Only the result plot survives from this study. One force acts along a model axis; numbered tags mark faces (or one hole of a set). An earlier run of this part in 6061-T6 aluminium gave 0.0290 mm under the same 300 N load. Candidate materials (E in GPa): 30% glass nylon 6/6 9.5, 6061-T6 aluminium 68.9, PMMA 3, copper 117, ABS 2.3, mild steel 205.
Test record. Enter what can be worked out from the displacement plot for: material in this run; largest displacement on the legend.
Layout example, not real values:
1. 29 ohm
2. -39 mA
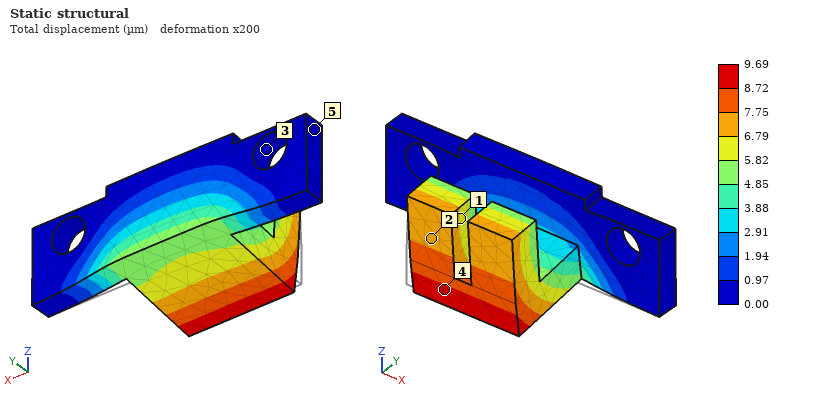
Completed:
1. mild steel
2. 9.69 µm
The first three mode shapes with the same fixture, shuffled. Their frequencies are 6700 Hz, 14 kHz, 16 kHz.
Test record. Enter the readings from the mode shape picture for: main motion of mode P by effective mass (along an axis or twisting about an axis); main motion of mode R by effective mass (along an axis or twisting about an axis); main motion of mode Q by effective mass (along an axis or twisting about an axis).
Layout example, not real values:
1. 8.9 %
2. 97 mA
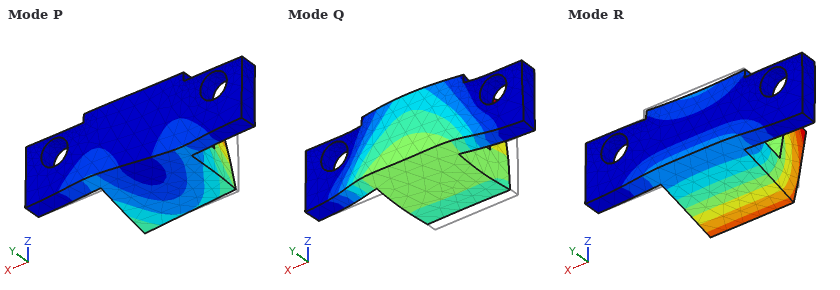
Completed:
1. along X
2. along Z
3. along Y
